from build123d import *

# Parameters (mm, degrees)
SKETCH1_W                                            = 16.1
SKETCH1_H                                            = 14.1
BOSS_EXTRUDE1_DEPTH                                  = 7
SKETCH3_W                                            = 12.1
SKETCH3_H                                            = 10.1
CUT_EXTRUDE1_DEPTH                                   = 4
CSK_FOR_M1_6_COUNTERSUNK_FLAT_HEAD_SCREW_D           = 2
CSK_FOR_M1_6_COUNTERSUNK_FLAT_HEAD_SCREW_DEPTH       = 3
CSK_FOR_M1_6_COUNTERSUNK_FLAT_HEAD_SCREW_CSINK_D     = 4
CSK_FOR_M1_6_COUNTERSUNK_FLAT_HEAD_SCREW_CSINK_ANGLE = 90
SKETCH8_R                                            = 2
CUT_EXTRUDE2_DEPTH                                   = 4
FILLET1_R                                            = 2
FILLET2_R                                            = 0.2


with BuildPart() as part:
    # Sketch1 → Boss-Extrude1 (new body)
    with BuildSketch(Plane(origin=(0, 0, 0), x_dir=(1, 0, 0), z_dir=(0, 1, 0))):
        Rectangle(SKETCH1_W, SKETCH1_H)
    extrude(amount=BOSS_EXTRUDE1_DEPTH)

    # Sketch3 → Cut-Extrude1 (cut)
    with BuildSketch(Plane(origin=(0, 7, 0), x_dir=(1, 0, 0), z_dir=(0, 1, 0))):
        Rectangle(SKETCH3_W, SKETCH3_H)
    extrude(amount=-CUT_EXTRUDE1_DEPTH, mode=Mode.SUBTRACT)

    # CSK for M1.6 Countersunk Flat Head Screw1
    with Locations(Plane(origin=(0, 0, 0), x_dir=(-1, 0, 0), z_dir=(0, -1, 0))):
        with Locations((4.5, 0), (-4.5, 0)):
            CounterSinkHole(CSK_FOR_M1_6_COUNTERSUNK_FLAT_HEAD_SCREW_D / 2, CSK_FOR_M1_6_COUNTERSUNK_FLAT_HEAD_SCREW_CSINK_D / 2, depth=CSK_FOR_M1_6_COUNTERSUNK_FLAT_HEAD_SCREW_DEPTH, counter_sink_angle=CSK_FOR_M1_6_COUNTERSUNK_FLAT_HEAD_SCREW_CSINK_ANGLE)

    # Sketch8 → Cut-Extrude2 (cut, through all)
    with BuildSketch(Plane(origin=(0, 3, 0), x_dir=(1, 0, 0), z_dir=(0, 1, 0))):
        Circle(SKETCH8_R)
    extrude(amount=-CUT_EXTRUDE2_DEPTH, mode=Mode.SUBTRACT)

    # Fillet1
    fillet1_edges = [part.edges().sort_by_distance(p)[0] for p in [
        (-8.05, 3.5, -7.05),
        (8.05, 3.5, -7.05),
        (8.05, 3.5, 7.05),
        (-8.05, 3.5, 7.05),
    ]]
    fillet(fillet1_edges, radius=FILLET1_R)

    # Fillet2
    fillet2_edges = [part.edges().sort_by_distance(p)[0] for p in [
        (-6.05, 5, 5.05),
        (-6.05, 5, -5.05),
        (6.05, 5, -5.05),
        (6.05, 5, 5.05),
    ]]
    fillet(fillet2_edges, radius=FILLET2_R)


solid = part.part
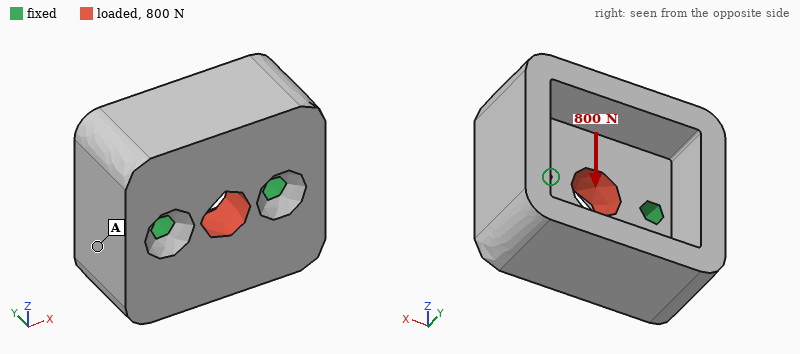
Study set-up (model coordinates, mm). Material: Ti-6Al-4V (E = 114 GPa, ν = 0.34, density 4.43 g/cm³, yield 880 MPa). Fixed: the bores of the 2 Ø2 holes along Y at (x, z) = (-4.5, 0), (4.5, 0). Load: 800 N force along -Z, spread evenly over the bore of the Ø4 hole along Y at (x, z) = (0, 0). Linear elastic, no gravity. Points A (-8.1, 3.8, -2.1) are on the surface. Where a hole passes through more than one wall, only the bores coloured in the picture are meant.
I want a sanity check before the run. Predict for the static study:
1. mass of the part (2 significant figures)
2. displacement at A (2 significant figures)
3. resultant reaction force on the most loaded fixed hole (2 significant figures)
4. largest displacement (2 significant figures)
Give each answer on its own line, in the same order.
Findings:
4.5 g
0.36 µm
400 N
1.6 µm
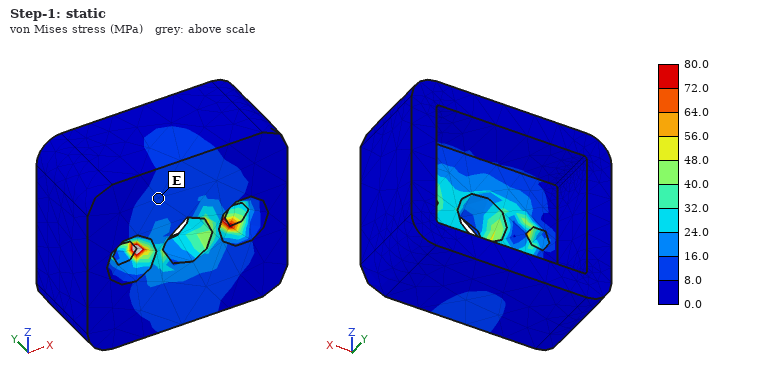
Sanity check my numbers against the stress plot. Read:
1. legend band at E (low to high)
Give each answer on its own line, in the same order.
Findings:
8.0 to 16.0 MPa
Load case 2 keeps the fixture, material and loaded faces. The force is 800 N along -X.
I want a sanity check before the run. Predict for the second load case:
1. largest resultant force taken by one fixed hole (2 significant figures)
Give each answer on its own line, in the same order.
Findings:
400 N
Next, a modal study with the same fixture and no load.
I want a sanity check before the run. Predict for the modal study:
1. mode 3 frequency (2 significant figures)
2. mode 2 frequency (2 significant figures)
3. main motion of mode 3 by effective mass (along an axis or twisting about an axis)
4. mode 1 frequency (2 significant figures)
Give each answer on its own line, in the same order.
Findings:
41 kHz
33 kHz
along Y
21 kHz
